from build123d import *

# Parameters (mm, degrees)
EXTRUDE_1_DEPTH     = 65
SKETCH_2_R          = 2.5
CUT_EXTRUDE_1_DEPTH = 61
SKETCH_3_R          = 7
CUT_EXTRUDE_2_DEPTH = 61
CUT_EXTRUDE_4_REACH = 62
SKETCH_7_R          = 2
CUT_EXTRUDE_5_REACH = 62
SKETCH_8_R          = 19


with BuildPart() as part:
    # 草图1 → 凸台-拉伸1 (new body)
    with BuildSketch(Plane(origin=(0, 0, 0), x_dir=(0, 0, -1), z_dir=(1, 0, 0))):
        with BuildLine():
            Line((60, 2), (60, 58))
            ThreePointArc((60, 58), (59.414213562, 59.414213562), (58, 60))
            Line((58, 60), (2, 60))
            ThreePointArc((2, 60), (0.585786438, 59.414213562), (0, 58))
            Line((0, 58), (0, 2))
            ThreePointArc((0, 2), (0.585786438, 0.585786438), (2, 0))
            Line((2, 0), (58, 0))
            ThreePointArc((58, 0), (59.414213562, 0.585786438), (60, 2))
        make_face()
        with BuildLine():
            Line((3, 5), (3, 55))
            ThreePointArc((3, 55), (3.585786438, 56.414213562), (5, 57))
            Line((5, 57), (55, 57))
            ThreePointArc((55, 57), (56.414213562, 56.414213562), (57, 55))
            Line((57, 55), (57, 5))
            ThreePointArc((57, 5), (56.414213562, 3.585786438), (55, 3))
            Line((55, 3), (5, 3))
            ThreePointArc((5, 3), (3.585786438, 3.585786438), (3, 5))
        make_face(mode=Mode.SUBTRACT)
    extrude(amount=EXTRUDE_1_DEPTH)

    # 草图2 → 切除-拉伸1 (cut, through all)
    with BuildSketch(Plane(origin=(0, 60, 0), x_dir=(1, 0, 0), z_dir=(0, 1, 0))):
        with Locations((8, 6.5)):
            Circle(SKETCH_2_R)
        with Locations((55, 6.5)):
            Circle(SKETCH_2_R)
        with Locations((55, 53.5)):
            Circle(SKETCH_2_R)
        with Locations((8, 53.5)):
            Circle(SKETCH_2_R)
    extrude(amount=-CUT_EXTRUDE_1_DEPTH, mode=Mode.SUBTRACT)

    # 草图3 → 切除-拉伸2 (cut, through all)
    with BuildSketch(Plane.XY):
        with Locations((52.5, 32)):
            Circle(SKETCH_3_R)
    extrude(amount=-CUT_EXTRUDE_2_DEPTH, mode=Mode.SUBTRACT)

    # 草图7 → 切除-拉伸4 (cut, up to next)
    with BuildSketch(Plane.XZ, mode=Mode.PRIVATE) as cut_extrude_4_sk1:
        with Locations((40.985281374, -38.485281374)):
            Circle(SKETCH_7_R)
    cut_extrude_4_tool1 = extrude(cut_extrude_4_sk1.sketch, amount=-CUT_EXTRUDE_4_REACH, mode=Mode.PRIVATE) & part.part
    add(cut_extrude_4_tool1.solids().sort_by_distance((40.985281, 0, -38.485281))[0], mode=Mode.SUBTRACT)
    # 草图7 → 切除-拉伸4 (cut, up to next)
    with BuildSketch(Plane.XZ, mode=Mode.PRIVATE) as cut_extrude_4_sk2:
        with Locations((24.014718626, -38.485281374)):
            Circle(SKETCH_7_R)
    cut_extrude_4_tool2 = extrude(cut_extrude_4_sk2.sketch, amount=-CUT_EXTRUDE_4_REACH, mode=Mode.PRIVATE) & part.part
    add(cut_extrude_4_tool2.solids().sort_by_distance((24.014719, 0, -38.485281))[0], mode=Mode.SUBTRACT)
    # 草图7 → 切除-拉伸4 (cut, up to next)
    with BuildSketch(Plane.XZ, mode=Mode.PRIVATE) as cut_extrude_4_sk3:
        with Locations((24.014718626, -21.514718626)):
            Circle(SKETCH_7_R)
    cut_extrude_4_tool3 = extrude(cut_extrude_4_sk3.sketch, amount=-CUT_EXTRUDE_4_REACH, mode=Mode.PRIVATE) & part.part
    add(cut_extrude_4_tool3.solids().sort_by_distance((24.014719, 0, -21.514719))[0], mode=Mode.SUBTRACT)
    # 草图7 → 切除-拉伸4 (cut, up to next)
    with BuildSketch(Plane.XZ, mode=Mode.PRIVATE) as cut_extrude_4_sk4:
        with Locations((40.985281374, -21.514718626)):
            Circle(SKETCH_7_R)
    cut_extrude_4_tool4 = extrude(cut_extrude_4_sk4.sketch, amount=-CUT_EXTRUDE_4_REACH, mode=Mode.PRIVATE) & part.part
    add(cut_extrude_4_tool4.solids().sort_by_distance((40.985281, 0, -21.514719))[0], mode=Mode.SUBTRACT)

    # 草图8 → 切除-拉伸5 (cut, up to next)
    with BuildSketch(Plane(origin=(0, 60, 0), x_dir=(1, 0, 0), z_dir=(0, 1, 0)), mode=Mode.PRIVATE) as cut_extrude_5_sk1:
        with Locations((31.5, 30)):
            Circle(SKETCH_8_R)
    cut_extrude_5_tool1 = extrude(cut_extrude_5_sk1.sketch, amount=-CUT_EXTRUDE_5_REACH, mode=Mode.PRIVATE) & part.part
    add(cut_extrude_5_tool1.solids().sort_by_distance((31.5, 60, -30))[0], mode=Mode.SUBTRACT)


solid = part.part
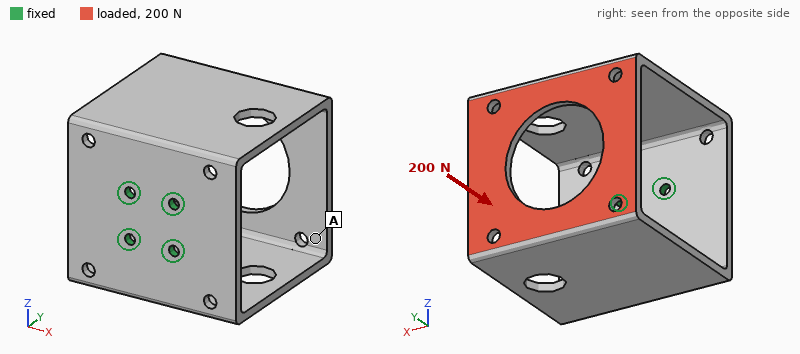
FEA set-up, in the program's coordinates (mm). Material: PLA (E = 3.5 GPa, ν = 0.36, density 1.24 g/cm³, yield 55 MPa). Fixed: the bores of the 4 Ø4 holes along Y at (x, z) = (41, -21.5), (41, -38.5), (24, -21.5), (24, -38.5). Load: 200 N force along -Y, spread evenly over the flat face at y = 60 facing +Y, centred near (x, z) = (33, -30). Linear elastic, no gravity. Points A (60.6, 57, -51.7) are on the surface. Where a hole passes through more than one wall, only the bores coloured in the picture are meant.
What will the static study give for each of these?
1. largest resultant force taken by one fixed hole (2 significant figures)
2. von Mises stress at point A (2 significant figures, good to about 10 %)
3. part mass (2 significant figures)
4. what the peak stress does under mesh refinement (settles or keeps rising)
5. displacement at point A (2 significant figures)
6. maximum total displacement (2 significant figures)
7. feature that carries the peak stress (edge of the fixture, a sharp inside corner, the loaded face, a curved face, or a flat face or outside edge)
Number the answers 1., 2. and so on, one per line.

1. 52 N
2. 2.8 MPa
3. 49 g
4. keeps rising
5. 0.70 mm
6. 1.2 mm
7. edge of the fixture
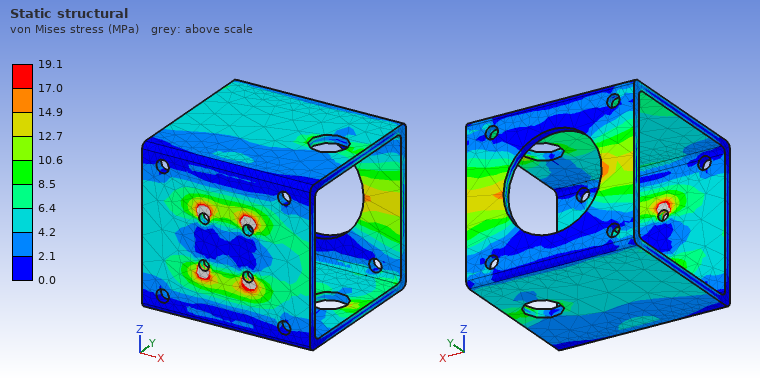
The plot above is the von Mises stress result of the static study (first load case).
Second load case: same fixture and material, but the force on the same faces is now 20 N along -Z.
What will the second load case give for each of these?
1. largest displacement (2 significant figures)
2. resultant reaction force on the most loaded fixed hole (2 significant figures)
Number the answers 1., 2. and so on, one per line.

1. 1.1 mm
2. 17 N
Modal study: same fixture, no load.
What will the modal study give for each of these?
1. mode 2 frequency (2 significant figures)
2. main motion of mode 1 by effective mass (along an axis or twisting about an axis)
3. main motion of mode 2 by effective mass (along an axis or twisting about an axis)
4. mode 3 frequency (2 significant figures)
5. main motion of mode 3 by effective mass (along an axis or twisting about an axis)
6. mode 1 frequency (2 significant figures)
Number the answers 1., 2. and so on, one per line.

1. 250 Hz
2. along Z
3. along X
4. 400 Hz
5. twisting about Y
6. 160 Hz
